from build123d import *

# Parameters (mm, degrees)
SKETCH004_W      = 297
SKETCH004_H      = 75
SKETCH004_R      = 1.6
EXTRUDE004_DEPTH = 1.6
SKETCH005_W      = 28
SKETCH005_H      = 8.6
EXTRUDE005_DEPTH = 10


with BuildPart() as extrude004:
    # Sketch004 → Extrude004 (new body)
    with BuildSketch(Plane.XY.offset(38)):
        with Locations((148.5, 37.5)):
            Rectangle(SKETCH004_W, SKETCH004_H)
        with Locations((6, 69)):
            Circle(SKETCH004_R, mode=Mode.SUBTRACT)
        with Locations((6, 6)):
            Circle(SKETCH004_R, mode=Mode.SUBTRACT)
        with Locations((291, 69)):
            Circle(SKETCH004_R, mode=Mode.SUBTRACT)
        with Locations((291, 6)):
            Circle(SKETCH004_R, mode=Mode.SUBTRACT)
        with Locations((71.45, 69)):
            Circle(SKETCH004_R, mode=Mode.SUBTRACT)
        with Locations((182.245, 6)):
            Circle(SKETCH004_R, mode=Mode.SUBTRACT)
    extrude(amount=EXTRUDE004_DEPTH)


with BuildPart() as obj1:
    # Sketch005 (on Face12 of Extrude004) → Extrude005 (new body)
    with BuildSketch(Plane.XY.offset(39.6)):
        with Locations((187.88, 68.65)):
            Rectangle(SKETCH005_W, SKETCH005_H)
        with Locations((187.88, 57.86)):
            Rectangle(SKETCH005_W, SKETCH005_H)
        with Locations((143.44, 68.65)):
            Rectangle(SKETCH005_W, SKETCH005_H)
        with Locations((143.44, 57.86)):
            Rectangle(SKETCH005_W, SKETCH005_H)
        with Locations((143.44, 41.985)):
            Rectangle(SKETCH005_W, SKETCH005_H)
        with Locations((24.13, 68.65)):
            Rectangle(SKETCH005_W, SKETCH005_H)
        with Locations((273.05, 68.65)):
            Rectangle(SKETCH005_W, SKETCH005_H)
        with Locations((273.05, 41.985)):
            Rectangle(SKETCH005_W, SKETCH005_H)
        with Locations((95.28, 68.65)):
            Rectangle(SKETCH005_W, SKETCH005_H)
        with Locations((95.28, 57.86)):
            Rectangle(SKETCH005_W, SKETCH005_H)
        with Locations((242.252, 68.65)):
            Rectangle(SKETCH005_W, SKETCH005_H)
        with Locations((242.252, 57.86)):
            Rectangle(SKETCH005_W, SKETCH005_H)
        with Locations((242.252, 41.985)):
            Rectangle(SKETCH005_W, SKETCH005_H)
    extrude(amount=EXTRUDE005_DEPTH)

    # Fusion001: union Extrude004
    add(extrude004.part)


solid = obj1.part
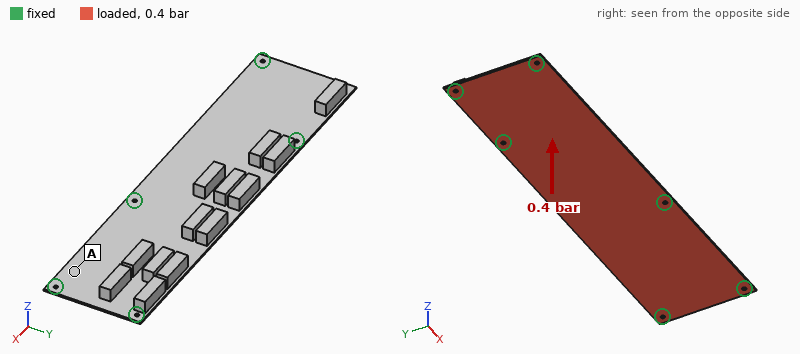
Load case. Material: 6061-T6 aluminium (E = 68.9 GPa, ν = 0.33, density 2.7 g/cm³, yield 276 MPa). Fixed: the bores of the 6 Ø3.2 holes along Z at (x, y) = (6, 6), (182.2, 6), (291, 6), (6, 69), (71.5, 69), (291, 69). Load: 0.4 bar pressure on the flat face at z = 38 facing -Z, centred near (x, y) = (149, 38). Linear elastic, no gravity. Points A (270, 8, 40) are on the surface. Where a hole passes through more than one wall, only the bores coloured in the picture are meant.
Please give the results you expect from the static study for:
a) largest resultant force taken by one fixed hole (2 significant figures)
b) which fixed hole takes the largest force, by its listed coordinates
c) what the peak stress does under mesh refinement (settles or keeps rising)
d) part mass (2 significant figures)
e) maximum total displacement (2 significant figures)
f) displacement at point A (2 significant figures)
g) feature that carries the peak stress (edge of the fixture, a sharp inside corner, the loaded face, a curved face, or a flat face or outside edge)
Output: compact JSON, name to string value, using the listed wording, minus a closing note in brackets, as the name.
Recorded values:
{"largest resultant force taken by one fixed hole": "320 N", "which fixed hole takes the largest force, by its listed coordinates": "(182.2, 6)", "what the peak stress does under mesh refinement": "keeps rising", "part mass": "180 g", "maximum total displacement": "1.8 mm", "displacement at point A": "0.28 mm", "feature that carries the peak stress": "edge of the fixture"}
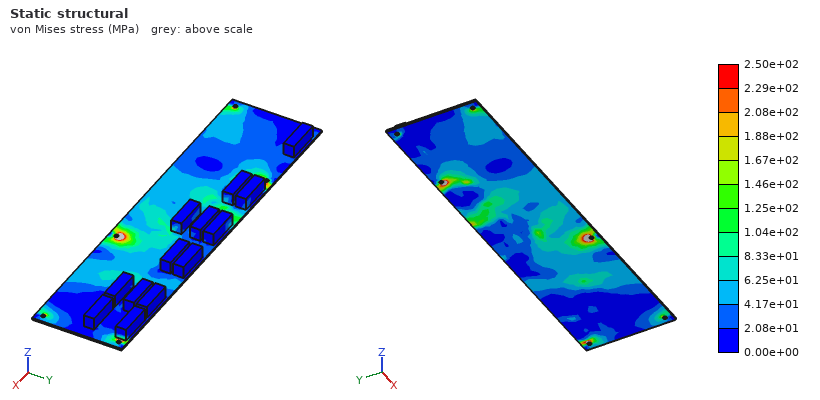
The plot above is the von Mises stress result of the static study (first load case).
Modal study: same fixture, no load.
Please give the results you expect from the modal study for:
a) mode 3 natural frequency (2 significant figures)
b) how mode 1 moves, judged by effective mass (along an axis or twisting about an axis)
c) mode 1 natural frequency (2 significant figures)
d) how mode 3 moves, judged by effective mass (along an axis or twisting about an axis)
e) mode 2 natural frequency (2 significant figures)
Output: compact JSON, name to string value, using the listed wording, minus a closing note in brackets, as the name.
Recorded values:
{"mode 3 natural frequency": "510 Hz", "how mode 1 moves, judged by effective mass": "along Z", "mode 1 natural frequency": "270 Hz", "how mode 3 moves, judged by effective mass": "along Z", "mode 2 natural frequency": "380 Hz"}
